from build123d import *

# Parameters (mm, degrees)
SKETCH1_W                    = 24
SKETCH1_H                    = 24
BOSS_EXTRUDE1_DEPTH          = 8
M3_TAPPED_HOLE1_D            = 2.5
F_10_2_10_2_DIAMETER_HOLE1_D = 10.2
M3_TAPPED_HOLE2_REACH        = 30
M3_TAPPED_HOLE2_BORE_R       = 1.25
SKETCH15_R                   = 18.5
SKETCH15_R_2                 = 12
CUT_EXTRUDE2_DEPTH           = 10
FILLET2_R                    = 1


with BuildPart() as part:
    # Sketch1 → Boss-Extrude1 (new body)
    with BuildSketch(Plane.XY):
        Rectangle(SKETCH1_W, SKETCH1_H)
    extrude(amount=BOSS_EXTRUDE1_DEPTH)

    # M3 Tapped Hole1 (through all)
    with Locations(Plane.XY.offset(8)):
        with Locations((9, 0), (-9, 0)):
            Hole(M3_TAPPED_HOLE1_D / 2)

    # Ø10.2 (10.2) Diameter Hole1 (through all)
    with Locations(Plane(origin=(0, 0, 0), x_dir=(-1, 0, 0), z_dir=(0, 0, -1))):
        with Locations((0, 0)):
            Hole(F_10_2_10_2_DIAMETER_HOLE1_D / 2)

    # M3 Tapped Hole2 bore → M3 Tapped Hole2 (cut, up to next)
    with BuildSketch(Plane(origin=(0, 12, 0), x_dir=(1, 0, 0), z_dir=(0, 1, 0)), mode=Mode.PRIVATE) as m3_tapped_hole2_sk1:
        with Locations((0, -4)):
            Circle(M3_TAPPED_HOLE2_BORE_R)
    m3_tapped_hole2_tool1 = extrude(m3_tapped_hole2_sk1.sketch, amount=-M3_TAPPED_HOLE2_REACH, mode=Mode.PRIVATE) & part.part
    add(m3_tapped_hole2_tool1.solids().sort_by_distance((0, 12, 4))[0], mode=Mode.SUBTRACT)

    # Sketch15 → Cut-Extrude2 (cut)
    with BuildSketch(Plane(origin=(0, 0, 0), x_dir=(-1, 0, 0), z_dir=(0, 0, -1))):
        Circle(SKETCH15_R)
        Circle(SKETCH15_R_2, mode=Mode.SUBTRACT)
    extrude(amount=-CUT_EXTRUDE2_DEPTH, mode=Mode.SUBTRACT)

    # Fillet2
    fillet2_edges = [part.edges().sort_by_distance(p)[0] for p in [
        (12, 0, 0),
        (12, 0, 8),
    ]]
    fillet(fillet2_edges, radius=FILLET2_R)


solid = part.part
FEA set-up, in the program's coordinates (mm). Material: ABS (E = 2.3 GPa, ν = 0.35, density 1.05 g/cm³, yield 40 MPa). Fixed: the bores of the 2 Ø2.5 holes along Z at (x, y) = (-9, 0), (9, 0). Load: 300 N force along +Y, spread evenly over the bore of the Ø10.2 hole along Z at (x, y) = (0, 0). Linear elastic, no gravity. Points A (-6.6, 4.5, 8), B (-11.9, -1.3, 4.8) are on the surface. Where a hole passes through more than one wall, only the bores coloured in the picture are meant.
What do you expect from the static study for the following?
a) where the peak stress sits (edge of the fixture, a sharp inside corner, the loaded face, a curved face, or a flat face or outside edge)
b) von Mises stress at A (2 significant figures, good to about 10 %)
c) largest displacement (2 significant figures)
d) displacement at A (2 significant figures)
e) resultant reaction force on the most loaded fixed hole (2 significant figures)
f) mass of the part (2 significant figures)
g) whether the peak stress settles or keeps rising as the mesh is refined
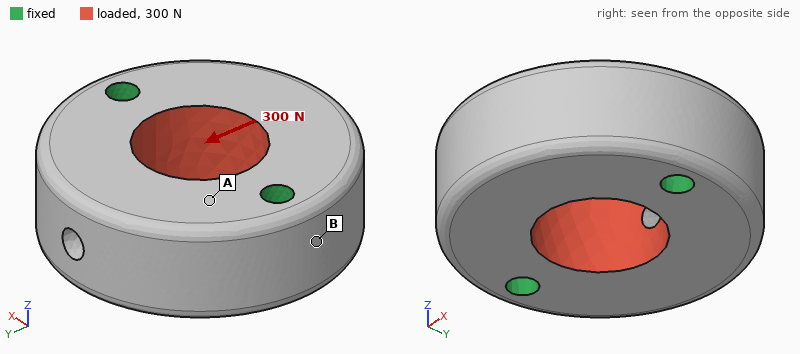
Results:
edge of the fixture
1.6 MPa
11 µm
4.8 µm
150 N
3.0 g
keeps rising
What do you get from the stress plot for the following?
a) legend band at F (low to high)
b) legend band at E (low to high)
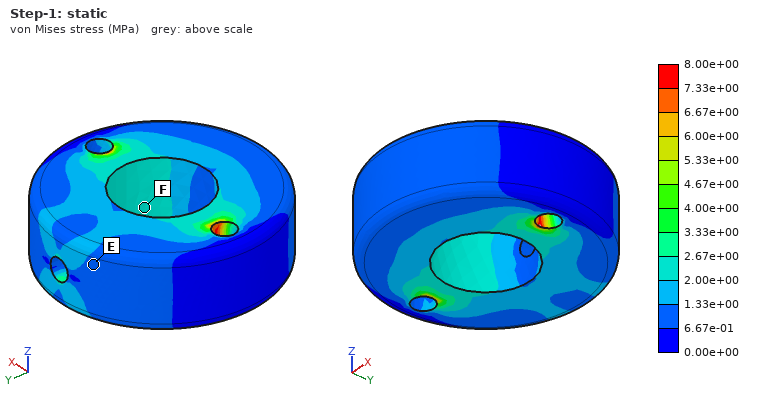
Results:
2.00e+00 to 2.67e+00 MPa
6.67e-01 to 1.33e+00 MPa
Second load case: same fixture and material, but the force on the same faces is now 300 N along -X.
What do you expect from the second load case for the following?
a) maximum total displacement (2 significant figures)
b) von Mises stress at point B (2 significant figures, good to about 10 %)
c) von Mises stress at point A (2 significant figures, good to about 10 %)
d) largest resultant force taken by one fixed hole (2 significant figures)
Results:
12 µm
2.0 MPa
1.5 MPa
150 N
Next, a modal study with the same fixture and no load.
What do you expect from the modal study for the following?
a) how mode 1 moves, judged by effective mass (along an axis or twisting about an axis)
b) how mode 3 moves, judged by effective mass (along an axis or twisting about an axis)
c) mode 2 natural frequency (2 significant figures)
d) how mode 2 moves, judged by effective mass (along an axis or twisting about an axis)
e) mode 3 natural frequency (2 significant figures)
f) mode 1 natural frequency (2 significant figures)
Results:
twisting about X
twisting about Z
10 kHz
along Z
15 kHz
9300 Hz
